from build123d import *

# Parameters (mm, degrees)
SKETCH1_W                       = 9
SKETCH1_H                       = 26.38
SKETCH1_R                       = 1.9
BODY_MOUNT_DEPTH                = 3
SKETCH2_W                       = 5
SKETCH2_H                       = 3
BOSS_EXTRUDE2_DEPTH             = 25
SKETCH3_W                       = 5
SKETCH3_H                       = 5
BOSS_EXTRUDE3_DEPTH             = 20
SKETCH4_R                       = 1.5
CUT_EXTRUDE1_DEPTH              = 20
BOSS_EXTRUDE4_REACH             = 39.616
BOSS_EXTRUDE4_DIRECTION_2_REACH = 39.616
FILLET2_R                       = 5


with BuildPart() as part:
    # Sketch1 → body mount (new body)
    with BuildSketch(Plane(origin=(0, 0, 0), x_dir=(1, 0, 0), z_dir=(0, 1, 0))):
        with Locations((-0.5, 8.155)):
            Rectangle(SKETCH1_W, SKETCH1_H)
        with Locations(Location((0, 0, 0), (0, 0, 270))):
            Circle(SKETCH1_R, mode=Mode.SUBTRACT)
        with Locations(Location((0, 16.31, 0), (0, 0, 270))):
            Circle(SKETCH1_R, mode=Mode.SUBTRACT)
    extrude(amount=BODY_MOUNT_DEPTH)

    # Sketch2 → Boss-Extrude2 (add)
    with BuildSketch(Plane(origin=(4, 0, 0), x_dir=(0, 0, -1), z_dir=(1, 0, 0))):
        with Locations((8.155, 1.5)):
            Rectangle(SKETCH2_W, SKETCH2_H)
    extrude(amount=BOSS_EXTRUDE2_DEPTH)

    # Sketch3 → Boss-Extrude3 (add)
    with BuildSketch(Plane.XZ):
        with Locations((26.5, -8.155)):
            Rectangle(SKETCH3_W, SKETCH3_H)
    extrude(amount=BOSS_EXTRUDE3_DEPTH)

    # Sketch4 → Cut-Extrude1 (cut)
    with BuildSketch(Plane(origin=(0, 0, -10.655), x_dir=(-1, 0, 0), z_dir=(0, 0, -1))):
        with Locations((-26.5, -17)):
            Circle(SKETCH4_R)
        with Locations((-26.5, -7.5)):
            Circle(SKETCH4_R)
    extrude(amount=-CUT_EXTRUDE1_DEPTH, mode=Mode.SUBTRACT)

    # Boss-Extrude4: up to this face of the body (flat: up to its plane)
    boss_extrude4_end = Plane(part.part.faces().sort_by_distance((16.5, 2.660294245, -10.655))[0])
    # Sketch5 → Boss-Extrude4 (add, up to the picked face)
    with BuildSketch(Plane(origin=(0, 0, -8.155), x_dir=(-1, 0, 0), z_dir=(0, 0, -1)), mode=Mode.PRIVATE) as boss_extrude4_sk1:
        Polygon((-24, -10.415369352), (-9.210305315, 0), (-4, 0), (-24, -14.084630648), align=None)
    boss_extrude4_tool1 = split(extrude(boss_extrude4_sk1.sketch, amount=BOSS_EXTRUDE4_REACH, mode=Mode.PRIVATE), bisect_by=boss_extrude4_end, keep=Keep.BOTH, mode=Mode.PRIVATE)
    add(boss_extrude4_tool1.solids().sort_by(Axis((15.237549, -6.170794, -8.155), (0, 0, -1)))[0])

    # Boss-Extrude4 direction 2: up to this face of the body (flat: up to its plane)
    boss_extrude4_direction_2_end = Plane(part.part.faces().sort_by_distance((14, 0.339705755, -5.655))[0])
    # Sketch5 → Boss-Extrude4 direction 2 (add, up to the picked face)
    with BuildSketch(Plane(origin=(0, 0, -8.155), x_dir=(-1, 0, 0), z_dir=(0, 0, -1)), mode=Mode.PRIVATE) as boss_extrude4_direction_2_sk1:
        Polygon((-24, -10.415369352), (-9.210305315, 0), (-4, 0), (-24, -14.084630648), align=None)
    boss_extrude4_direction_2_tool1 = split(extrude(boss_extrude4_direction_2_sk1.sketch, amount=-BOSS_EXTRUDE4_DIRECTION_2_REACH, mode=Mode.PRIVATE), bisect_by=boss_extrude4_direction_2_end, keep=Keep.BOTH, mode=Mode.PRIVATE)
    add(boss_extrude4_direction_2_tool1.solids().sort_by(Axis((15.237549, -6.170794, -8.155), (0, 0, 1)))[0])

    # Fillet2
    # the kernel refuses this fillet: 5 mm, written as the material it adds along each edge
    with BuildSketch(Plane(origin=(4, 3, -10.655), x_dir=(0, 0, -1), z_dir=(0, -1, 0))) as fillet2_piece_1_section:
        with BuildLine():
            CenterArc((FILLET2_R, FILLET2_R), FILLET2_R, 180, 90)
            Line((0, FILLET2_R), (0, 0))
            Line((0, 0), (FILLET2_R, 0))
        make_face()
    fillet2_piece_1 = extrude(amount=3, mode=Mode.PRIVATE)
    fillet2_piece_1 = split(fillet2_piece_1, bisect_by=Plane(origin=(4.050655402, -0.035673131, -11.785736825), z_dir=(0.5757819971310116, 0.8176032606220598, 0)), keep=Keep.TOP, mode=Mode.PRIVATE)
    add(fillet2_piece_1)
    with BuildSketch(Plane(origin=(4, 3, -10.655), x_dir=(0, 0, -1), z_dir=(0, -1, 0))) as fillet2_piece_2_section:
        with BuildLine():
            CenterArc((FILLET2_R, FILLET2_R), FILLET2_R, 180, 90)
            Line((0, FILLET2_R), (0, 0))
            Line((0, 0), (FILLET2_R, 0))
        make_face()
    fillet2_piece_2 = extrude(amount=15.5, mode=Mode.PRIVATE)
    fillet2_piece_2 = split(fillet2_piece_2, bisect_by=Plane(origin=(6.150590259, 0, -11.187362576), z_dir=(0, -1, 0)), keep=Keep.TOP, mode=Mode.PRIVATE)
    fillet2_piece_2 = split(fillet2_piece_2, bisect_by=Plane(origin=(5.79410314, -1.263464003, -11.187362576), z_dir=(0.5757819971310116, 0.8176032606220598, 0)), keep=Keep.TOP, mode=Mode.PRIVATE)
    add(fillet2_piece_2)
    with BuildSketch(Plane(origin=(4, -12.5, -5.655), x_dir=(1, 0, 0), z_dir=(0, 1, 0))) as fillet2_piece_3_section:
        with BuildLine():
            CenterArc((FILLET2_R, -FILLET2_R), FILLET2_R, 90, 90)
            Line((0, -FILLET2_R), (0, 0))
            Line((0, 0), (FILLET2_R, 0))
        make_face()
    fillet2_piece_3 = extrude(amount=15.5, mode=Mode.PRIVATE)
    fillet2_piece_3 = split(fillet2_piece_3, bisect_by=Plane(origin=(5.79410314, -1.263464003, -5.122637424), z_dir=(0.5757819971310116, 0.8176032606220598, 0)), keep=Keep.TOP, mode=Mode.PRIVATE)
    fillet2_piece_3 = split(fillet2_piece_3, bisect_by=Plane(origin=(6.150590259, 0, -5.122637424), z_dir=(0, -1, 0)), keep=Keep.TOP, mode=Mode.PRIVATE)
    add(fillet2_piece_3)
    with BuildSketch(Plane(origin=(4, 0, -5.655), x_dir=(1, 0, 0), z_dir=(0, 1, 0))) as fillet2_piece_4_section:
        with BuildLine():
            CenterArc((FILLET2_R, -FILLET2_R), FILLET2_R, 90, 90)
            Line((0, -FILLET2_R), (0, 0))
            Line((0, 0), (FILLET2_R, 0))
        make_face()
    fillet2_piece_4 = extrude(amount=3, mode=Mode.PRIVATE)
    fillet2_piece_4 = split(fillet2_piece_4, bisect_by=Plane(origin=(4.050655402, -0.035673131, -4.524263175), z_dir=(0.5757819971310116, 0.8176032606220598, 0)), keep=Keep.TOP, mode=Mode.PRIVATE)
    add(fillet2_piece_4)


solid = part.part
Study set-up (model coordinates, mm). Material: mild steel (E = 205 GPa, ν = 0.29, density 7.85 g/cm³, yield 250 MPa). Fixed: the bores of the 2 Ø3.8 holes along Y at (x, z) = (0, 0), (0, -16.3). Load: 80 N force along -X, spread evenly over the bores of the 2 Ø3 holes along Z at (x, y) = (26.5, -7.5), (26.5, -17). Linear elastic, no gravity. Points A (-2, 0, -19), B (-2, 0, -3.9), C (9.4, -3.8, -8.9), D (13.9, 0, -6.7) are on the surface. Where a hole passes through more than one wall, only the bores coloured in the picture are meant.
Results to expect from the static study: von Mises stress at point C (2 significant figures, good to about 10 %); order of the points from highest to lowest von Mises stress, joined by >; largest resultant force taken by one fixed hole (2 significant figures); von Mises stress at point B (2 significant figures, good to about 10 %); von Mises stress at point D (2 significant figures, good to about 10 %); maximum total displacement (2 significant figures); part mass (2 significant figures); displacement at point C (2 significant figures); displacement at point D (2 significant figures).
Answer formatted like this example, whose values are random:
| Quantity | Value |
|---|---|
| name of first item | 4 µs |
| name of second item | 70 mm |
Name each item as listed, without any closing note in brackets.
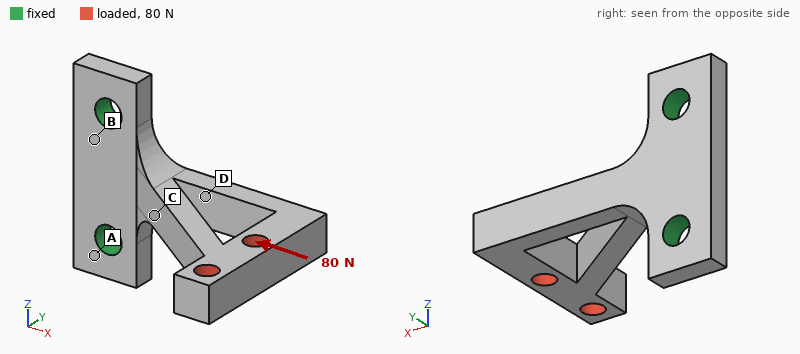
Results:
| Quantity | Value |
|---|---|
| von Mises stress at point C | 46 MPa |
| order of the points from highest to lowest von Mises stress, joined by > | C > D > B > A |
| largest resultant force taken by one fixed hole | 42 N |
| von Mises stress at point B | 16 MPa |
| von Mises stress at point D | 29 MPa |
| maximum total displacement | 78 µm |
| part mass | 14 g |
| displacement at point C | 14 µm |
| displacement at point D | 20 µm |
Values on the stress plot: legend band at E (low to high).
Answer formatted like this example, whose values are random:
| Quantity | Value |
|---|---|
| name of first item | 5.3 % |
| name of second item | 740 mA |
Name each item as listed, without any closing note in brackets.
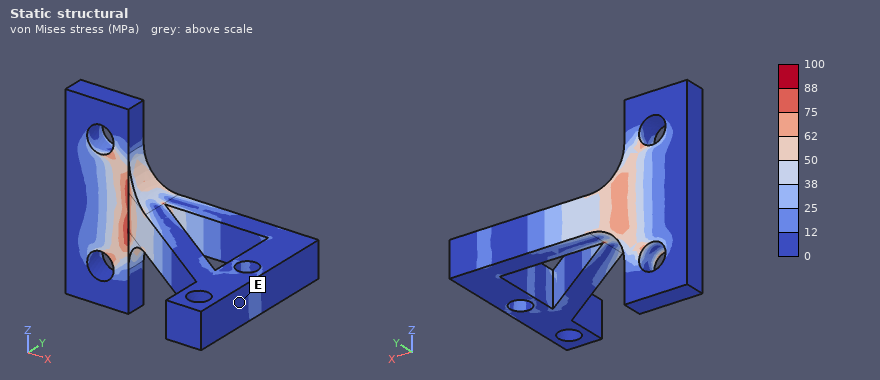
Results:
| Quantity | Value |
|---|---|
| legend band at E | 0 to 12 MPa |
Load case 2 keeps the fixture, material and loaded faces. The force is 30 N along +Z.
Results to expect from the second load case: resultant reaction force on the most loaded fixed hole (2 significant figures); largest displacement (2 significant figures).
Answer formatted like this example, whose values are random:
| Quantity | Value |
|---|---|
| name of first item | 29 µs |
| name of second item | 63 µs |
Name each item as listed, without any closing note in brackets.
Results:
| Quantity | Value |
|---|---|
| resultant reaction force on the most loaded fixed hole | 66 N |
| largest displacement | 25 µm |
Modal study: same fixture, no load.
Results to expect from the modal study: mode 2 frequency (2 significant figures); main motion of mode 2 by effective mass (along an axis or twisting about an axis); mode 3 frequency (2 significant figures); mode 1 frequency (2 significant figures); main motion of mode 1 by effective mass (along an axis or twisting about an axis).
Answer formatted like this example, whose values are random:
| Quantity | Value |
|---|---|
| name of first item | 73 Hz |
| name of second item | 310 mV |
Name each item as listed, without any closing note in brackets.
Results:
| Quantity | Value |
|---|---|
| mode 2 frequency | 3500 Hz |
| main motion of mode 2 by effective mass | along Z |
| mode 3 frequency | 7100 Hz |
| mode 1 frequency | 1900 Hz |
| main motion of mode 1 by effective mass | along Y |
